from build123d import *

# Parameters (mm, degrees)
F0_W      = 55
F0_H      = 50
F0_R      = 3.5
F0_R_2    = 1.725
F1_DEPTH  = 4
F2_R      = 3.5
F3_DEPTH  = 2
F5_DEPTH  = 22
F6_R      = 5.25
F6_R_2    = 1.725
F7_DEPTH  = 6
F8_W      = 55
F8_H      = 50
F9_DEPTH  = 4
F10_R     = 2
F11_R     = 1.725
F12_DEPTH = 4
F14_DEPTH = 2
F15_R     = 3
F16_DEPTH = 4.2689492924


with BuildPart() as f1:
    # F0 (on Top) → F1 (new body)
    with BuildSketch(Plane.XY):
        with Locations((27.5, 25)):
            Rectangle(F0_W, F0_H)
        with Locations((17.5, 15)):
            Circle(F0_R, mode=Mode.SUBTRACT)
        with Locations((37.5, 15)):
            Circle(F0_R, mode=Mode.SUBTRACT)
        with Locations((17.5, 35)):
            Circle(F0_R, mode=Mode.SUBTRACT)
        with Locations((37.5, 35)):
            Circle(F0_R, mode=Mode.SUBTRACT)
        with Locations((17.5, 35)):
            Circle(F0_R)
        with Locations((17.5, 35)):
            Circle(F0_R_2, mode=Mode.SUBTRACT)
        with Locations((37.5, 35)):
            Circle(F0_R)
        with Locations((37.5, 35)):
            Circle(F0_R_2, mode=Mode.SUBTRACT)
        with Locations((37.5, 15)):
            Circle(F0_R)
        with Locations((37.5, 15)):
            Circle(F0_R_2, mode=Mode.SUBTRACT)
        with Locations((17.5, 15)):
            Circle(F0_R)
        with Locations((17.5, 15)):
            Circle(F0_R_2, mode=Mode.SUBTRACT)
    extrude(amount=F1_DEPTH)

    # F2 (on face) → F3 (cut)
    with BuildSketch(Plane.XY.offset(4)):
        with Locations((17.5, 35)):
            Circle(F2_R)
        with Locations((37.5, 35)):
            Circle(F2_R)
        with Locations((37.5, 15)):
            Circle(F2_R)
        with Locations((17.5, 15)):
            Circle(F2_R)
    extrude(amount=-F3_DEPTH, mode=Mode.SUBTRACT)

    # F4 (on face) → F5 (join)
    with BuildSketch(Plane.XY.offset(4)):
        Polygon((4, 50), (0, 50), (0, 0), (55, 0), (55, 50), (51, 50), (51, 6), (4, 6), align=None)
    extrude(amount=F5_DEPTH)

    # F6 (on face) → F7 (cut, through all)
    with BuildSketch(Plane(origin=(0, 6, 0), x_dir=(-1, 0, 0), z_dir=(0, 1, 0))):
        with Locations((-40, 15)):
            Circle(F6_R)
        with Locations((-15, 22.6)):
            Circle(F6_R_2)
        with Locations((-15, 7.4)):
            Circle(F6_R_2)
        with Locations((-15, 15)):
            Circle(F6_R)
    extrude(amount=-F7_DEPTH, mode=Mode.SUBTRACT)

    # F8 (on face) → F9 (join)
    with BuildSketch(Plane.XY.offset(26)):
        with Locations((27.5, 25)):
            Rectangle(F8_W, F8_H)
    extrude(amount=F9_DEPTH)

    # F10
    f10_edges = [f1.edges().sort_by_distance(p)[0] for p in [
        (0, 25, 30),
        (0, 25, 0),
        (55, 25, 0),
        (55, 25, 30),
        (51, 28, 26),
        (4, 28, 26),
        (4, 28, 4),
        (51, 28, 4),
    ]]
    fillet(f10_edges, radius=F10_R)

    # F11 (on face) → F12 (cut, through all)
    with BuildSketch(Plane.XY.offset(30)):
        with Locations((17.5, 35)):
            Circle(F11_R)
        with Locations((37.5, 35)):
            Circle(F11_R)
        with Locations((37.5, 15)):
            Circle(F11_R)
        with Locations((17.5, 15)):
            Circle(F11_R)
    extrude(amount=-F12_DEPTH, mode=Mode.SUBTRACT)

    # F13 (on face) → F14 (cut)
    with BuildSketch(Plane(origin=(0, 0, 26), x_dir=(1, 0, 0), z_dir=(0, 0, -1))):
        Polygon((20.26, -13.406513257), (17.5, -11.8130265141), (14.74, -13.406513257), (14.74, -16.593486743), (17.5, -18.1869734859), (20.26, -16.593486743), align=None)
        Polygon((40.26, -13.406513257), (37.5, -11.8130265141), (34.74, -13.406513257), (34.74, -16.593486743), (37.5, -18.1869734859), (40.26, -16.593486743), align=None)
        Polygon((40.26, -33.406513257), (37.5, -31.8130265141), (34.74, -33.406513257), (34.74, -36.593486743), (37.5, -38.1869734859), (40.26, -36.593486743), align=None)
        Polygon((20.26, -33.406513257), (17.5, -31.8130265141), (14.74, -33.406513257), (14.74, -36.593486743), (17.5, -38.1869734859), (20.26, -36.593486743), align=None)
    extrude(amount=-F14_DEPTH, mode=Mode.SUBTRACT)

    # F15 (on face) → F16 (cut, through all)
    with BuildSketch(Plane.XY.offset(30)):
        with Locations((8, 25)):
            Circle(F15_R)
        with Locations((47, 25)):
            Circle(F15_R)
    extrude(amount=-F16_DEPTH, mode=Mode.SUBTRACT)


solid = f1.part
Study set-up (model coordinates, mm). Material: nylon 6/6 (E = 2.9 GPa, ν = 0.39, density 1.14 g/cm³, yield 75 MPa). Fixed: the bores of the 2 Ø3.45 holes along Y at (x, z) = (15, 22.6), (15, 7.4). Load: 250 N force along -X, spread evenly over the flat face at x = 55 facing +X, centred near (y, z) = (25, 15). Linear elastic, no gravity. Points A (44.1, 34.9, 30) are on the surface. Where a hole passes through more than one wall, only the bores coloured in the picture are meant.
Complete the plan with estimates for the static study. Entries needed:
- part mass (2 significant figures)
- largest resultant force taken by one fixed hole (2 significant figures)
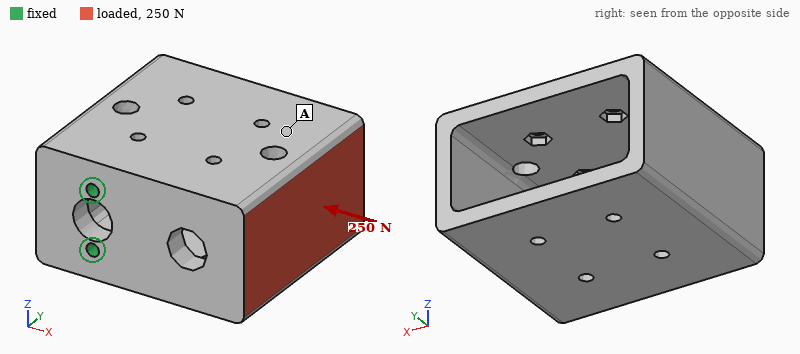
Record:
40 g
130 N
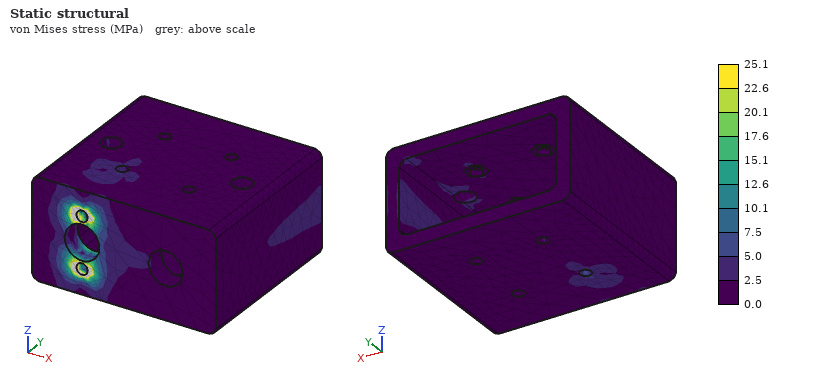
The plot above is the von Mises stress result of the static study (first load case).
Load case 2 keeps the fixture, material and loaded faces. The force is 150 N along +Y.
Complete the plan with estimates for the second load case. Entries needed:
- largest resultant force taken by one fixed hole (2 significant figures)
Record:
75 N
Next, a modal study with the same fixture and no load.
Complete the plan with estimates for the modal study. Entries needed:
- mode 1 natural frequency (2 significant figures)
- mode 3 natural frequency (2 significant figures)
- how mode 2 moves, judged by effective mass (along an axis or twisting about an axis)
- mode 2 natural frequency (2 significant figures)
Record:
510 Hz
1500 Hz
along Z
830 Hz
